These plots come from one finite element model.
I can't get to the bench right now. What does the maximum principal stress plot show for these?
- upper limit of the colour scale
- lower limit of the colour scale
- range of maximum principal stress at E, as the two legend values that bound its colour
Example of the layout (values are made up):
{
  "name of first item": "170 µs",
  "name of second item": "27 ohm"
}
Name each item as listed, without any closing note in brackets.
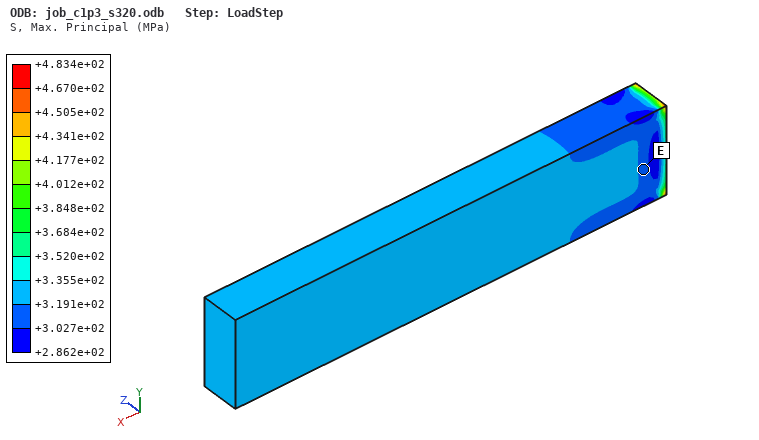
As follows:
{
  "upper limit of the colour scale": "+4.834e+02 MPa",
  "lower limit of the colour scale": "+2.862e+02 MPa",
  "range of maximum principal stress at E, as the two legend values that bound its colour": "+3.027e+02 to +3.191e+02 MPa"
}
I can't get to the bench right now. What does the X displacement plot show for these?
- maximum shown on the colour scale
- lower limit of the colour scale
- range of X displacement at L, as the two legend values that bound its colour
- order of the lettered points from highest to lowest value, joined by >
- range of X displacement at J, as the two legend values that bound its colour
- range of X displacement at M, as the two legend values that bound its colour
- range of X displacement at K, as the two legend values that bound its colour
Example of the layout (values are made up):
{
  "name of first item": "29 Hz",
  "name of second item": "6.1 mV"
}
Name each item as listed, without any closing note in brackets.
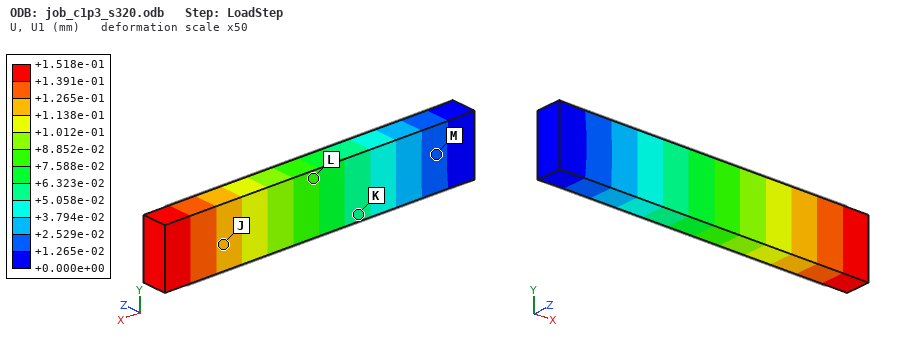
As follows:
{
  "maximum shown on the colour scale": "+1.518e-01 mm",
  "lower limit of the colour scale": "+0.000e+00 mm",
  "range of X displacement at L, as the two legend values that bound its colour": "+7.588e-02 to +8.852e-02 mm",
  "order of the lettered points from highest to lowest value, joined by >": "J > L > K > M",
  "range of X displacement at J, as the two legend values that bound its colour": "+1.138e-01 to +1.265e-01 mm",
  "range of X displacement at M, as the two legend values that bound its colour": "+1.265e-02 to +2.529e-02 mm",
  "range of X displacement at K, as the two legend values that bound its colour": "+5.058e-02 to +6.323e-02 mm"
}
